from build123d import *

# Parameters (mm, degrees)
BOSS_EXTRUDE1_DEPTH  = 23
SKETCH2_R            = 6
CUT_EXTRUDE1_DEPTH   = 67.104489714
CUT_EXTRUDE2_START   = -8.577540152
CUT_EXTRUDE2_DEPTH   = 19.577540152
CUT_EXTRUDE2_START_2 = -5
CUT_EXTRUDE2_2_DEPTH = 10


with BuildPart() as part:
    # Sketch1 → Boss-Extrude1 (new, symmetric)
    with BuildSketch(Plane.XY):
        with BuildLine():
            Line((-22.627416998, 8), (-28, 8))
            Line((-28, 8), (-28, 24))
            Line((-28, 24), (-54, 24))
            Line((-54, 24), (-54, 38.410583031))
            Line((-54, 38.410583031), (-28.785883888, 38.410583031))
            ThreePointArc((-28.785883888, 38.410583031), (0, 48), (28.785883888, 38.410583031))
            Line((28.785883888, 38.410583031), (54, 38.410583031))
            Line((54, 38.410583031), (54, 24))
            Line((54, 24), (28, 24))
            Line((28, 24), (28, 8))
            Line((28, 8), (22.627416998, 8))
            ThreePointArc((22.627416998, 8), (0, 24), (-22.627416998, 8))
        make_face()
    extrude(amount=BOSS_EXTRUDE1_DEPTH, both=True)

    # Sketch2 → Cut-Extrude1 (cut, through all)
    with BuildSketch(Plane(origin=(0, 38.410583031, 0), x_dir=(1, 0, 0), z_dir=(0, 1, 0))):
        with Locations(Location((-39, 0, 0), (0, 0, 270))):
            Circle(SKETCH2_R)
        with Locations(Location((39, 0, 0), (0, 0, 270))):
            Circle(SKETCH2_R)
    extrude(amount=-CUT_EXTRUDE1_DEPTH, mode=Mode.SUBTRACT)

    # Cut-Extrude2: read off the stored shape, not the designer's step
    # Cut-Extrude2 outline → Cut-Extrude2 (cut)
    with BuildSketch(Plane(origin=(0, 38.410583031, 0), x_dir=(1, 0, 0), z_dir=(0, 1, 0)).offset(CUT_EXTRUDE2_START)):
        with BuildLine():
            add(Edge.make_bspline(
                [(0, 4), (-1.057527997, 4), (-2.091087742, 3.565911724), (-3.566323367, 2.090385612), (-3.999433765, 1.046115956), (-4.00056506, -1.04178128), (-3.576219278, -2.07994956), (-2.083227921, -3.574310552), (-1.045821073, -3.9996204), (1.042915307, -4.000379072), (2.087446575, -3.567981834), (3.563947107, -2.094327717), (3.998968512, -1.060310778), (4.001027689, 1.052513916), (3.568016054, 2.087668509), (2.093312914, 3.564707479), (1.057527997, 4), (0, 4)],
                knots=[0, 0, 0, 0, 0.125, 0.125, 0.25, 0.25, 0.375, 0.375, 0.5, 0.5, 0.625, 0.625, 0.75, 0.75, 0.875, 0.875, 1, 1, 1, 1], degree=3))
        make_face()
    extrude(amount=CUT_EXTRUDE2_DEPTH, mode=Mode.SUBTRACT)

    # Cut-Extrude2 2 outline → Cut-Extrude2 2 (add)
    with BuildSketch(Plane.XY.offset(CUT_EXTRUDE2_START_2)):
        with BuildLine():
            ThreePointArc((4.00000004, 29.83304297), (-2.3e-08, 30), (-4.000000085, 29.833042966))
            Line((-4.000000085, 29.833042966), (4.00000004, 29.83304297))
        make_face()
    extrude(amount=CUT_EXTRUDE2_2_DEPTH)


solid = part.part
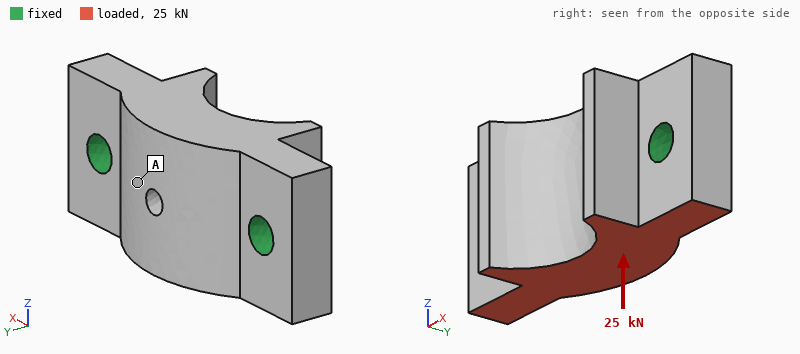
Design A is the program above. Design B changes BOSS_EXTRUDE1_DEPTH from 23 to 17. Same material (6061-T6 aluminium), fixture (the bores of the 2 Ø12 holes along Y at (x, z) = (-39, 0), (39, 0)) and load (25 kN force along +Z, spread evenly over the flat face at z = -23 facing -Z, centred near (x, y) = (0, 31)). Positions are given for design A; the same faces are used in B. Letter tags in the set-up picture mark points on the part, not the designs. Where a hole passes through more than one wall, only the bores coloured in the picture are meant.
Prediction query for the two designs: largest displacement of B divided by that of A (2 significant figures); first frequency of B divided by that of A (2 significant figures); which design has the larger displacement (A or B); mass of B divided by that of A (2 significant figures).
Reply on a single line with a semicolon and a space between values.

1.4; 1.2; B; 0.73
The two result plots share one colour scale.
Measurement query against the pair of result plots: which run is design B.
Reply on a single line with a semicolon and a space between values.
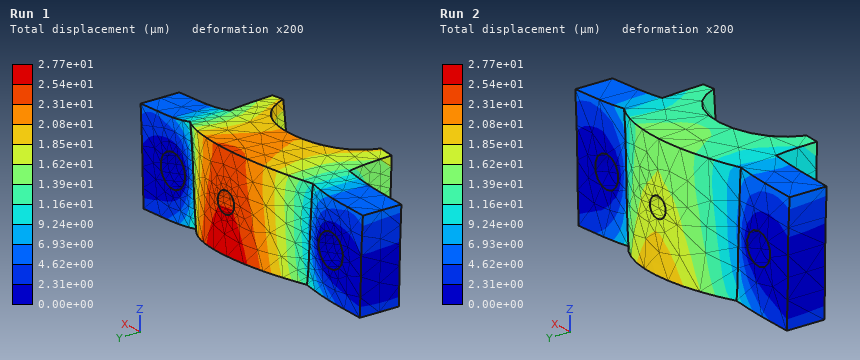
Run 1
